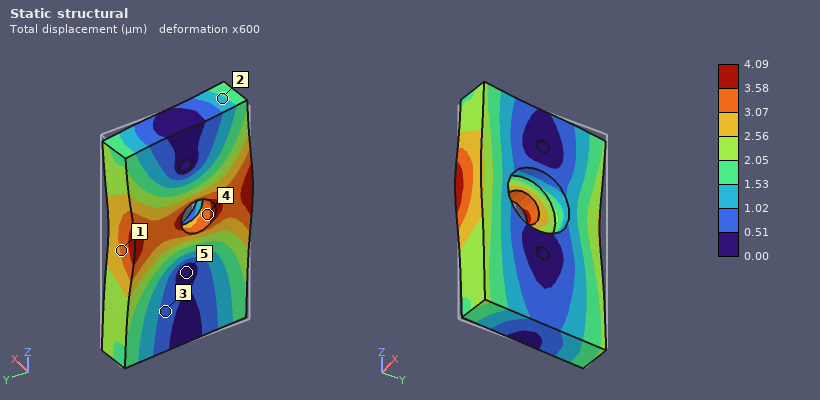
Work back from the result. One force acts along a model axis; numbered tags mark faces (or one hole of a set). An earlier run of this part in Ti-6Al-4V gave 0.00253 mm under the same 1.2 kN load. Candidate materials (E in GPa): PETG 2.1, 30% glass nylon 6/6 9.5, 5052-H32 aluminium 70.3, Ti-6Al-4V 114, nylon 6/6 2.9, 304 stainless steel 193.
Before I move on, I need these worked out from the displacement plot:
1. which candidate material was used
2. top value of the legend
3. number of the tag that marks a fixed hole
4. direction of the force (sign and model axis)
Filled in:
5052-H32 aluminium
4.09 µm
5
-Y
